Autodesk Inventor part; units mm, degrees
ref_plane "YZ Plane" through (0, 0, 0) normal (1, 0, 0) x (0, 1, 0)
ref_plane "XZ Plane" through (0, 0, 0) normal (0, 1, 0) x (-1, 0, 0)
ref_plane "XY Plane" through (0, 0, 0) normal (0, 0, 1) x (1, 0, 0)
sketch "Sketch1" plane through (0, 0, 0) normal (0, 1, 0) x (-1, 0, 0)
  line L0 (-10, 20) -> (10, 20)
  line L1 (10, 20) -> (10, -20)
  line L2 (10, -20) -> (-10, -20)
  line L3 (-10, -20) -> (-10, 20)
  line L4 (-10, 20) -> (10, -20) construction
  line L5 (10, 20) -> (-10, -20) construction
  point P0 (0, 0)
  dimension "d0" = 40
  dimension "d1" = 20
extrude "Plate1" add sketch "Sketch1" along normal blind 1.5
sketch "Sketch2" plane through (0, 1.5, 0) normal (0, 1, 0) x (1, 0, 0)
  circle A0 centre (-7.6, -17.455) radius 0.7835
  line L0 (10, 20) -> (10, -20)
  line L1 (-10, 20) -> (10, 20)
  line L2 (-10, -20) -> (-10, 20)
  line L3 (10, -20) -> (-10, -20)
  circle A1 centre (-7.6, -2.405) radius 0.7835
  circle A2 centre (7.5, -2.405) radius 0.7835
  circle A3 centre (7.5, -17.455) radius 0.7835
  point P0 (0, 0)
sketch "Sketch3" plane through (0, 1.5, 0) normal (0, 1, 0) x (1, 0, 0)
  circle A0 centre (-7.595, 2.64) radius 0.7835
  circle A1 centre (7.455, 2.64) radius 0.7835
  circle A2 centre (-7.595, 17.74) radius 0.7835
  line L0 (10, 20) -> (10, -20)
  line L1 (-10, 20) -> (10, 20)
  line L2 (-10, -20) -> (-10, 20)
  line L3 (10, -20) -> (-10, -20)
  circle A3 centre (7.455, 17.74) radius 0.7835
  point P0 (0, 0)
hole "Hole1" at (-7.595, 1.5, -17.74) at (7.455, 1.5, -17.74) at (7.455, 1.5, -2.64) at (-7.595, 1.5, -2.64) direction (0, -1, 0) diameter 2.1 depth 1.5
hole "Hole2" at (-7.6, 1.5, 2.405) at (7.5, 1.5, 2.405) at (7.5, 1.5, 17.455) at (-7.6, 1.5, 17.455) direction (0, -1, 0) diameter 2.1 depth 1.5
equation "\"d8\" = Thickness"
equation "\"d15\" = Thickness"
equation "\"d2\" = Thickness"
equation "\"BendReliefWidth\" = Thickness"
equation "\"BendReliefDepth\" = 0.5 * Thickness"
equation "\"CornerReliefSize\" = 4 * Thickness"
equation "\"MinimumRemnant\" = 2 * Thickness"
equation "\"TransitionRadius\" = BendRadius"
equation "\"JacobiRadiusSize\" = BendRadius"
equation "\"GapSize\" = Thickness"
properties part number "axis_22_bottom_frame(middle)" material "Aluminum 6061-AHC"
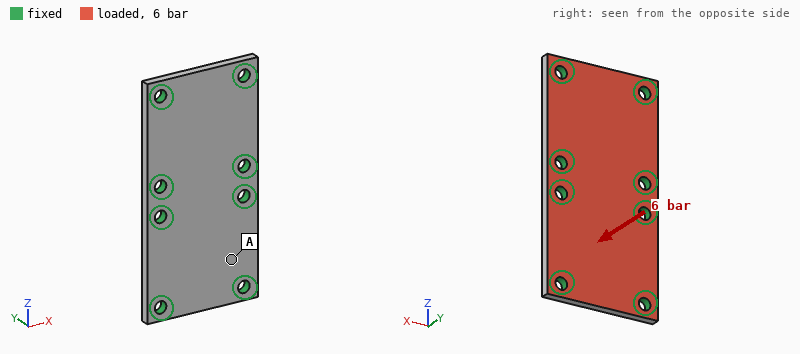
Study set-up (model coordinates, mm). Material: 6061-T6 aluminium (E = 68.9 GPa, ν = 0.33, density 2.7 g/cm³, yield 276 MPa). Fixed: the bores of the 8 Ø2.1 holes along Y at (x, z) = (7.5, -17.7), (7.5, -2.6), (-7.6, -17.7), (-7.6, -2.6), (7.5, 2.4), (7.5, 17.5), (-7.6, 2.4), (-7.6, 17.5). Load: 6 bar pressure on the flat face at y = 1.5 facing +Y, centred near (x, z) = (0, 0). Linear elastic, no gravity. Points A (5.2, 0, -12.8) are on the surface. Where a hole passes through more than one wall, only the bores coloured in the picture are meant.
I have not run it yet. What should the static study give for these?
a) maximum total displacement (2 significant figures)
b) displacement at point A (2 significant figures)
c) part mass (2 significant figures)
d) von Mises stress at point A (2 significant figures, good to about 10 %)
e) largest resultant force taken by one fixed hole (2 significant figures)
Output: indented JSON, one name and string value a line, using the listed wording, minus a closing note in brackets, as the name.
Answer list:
{
  "maximum total displacement": "8.1 µm",
  "displacement at point A": "4.9 µm",
  "part mass": "3.1 g",
  "von Mises stress at point A": "10 MPa",
  "largest resultant force taken by one fixed hole": "59 N"
}
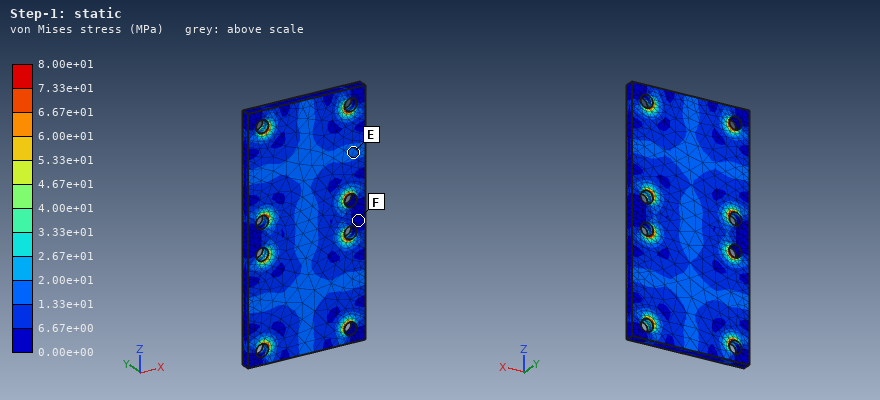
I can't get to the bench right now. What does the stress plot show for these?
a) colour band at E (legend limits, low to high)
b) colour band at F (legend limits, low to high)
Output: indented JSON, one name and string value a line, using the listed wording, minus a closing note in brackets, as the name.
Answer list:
{
  "colour band at E": "1.33e+01 to 2.00e+01 MPa",
  "colour band at F": "0.00e+00 to 6.67e+00 MPa"
}
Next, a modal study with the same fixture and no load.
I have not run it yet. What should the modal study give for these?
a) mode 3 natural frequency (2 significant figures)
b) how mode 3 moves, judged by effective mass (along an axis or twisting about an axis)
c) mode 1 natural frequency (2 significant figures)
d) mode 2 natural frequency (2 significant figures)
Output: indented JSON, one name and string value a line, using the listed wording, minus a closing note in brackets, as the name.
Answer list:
{
  "mode 3 natural frequency": "40 kHz",
  "how mode 3 moves, judged by effective mass": "twisting about Z",
  "mode 1 natural frequency": "26 kHz",
  "mode 2 natural frequency": "26 kHz"
}
